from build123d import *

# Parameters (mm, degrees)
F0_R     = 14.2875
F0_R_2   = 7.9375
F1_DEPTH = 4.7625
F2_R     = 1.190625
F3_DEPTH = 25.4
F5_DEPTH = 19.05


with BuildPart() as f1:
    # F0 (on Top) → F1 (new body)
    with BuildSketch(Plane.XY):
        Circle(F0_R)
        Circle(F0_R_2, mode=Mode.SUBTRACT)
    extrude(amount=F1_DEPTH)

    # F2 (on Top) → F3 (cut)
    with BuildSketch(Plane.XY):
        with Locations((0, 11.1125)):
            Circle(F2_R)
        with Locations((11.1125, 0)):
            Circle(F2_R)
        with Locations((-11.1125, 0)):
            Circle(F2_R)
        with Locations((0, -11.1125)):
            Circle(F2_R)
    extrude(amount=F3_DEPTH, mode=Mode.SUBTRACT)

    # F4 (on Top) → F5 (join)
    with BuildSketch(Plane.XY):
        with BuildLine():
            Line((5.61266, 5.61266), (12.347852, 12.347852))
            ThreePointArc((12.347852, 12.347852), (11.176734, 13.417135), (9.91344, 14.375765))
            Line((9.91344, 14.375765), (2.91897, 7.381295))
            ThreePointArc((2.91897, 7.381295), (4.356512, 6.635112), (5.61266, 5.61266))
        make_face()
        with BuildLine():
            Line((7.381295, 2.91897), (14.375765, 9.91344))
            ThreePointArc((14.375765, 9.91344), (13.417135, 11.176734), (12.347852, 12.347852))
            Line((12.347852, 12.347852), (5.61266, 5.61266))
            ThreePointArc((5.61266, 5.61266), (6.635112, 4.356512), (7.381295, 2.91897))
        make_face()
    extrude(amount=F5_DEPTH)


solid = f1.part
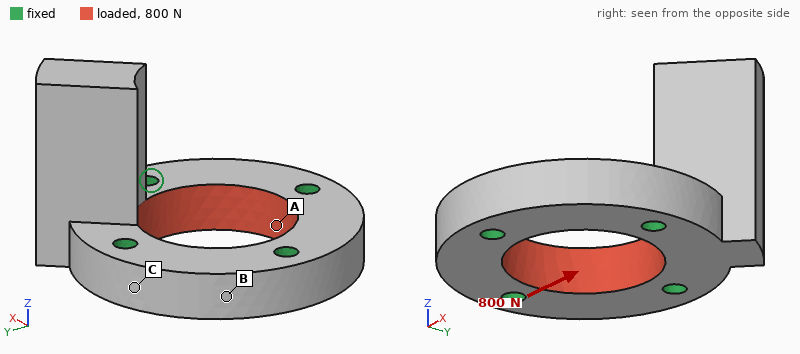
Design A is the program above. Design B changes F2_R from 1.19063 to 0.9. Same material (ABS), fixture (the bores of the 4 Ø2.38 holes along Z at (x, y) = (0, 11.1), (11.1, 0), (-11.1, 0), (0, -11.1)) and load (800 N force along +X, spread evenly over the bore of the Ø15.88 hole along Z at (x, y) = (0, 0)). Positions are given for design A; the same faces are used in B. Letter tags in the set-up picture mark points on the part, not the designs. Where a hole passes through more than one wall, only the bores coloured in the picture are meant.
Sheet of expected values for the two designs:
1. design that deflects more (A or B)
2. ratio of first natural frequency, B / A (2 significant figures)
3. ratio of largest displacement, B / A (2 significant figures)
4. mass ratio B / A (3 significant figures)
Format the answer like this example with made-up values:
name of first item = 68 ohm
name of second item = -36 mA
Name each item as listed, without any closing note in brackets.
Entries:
design that deflects more = B
ratio of first natural frequency, B / A = 0.96
ratio of largest displacement, B / A = 1.1
mass ratio B / A = 1.01
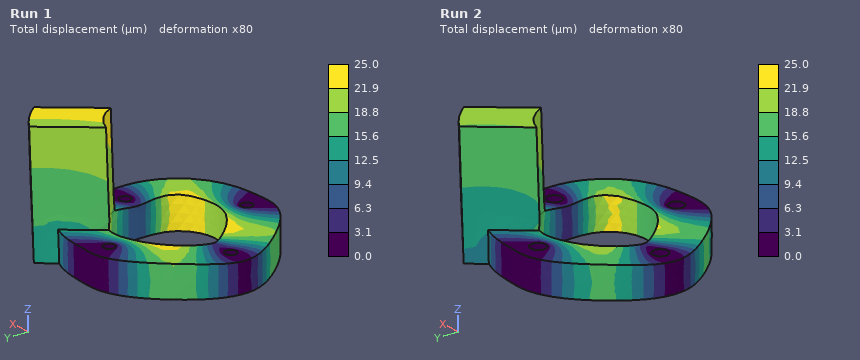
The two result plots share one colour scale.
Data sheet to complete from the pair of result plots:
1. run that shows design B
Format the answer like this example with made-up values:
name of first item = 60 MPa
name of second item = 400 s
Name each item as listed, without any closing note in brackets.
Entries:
run that shows design B = Run 1
